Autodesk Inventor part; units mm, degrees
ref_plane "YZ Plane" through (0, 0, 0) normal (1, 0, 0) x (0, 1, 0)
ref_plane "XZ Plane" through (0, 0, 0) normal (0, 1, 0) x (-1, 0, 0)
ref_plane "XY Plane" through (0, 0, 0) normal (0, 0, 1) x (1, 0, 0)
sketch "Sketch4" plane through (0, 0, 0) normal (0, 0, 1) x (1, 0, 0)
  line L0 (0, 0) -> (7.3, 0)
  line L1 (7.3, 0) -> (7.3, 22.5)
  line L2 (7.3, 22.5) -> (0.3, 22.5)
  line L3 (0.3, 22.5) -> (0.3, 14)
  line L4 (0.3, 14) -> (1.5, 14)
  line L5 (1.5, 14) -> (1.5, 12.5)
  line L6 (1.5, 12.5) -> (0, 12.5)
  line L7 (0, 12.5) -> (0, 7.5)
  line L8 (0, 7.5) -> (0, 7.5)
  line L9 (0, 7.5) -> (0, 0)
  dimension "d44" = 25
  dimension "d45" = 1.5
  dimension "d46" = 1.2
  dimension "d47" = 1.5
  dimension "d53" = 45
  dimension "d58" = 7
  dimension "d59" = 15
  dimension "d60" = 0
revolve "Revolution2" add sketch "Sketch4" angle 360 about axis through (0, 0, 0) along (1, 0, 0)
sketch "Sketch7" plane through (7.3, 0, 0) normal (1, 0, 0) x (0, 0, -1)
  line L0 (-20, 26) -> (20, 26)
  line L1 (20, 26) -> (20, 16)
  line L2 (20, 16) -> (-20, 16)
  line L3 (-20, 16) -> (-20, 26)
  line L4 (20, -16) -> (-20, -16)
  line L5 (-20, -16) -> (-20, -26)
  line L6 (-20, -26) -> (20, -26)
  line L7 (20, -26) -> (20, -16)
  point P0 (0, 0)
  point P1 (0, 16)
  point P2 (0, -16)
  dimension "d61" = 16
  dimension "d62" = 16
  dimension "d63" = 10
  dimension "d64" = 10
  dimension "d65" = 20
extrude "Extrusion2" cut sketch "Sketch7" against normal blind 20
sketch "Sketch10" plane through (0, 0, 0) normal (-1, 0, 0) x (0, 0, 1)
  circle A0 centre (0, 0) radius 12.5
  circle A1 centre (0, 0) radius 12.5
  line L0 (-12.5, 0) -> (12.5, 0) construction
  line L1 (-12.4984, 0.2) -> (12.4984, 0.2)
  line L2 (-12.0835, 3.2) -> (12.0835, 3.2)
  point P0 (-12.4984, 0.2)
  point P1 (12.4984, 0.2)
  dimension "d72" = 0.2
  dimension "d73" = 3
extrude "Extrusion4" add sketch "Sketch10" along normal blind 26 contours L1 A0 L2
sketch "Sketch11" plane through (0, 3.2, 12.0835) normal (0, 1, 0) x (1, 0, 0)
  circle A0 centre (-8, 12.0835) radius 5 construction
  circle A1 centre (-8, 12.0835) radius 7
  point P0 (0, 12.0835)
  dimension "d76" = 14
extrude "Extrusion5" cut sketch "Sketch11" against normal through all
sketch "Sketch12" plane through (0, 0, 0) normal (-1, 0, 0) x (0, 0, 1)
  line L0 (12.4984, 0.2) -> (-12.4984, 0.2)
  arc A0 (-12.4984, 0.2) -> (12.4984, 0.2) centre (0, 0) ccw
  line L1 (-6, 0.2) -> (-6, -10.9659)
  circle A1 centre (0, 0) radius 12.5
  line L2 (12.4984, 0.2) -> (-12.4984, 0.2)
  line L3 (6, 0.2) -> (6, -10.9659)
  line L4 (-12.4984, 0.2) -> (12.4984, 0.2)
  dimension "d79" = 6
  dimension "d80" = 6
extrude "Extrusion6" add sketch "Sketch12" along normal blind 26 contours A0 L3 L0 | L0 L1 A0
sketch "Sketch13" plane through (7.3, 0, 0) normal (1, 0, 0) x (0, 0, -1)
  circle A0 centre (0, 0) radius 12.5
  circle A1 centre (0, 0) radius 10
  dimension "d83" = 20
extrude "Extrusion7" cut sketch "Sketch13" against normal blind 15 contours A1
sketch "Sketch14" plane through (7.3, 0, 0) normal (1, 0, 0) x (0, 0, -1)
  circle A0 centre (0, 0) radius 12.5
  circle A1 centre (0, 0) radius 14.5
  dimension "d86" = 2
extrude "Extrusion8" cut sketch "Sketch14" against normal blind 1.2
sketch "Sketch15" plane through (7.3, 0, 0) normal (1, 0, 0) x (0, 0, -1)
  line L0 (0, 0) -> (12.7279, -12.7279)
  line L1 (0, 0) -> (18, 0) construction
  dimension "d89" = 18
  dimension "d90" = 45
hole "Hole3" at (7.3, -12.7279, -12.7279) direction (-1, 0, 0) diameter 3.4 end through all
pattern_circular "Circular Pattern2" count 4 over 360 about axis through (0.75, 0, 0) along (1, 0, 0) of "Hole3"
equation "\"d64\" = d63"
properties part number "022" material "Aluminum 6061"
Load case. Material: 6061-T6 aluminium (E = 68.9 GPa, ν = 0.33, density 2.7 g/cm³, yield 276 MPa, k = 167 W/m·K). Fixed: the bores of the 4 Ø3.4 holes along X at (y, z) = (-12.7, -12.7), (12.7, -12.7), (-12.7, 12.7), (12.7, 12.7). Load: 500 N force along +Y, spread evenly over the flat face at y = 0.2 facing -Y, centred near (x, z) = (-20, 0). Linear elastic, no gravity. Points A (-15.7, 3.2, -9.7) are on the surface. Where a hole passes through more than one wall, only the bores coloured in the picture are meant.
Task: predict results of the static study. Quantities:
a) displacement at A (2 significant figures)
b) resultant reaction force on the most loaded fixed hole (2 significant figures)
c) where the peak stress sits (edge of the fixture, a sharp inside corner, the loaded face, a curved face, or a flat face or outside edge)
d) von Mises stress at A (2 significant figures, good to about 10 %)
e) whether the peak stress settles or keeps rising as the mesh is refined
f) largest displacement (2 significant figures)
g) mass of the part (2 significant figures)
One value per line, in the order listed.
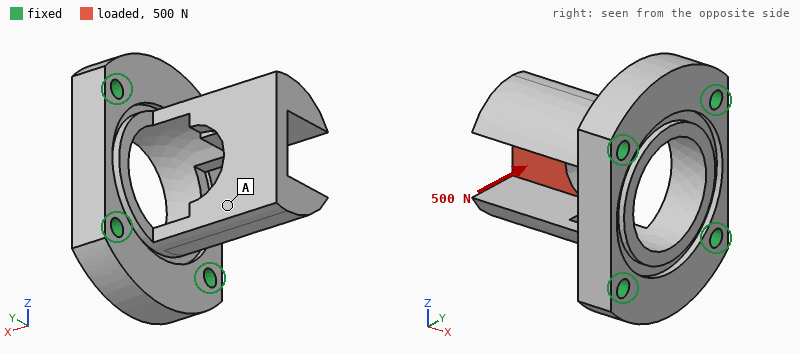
39 µm
330 N
a sharp inside corner
14 MPa
keeps rising
84 µm
27 g
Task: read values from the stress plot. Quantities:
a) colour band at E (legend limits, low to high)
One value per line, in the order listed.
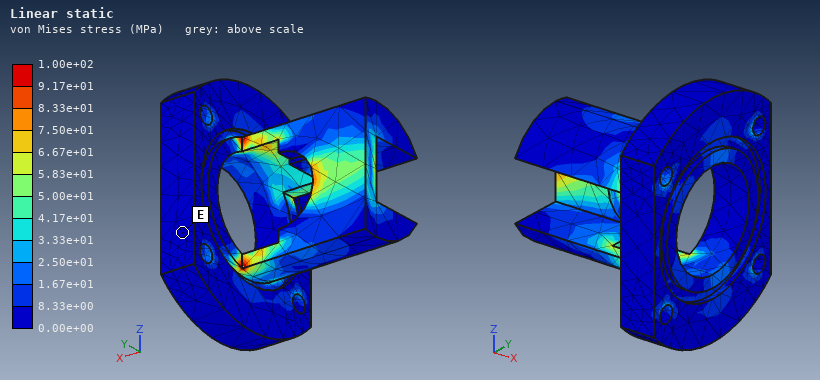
0.00e+00 to 8.33e+00 MPa
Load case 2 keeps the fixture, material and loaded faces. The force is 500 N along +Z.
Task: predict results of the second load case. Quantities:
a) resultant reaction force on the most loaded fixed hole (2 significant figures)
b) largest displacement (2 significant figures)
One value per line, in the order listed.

310 N
52 µm
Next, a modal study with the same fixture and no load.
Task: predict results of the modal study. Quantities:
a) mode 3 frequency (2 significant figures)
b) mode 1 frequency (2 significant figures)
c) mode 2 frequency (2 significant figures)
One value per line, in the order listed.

10 kHz
6200 Hz
6300 Hz
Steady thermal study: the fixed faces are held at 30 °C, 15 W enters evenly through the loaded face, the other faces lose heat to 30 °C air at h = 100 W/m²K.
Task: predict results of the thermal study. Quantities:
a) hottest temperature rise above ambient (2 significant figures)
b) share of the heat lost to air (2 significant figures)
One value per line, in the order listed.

24 K
24 %
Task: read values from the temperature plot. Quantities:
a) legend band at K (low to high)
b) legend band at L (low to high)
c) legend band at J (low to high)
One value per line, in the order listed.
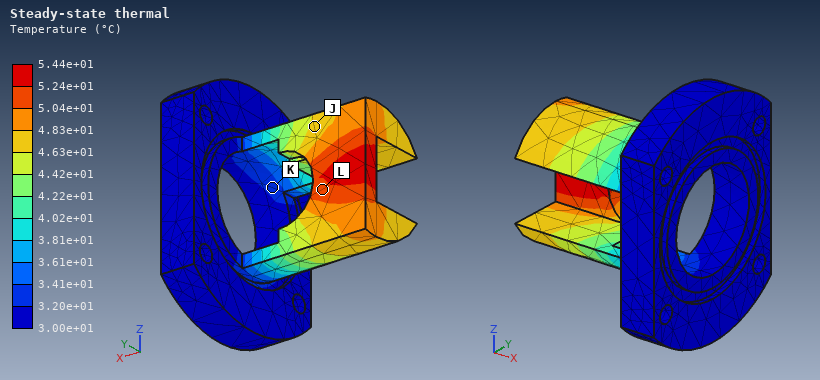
3.20e+01 to 3.41e+01 °C
5.04e+01 to 5.24e+01 °C
4.63e+01 to 4.83e+01 °C
